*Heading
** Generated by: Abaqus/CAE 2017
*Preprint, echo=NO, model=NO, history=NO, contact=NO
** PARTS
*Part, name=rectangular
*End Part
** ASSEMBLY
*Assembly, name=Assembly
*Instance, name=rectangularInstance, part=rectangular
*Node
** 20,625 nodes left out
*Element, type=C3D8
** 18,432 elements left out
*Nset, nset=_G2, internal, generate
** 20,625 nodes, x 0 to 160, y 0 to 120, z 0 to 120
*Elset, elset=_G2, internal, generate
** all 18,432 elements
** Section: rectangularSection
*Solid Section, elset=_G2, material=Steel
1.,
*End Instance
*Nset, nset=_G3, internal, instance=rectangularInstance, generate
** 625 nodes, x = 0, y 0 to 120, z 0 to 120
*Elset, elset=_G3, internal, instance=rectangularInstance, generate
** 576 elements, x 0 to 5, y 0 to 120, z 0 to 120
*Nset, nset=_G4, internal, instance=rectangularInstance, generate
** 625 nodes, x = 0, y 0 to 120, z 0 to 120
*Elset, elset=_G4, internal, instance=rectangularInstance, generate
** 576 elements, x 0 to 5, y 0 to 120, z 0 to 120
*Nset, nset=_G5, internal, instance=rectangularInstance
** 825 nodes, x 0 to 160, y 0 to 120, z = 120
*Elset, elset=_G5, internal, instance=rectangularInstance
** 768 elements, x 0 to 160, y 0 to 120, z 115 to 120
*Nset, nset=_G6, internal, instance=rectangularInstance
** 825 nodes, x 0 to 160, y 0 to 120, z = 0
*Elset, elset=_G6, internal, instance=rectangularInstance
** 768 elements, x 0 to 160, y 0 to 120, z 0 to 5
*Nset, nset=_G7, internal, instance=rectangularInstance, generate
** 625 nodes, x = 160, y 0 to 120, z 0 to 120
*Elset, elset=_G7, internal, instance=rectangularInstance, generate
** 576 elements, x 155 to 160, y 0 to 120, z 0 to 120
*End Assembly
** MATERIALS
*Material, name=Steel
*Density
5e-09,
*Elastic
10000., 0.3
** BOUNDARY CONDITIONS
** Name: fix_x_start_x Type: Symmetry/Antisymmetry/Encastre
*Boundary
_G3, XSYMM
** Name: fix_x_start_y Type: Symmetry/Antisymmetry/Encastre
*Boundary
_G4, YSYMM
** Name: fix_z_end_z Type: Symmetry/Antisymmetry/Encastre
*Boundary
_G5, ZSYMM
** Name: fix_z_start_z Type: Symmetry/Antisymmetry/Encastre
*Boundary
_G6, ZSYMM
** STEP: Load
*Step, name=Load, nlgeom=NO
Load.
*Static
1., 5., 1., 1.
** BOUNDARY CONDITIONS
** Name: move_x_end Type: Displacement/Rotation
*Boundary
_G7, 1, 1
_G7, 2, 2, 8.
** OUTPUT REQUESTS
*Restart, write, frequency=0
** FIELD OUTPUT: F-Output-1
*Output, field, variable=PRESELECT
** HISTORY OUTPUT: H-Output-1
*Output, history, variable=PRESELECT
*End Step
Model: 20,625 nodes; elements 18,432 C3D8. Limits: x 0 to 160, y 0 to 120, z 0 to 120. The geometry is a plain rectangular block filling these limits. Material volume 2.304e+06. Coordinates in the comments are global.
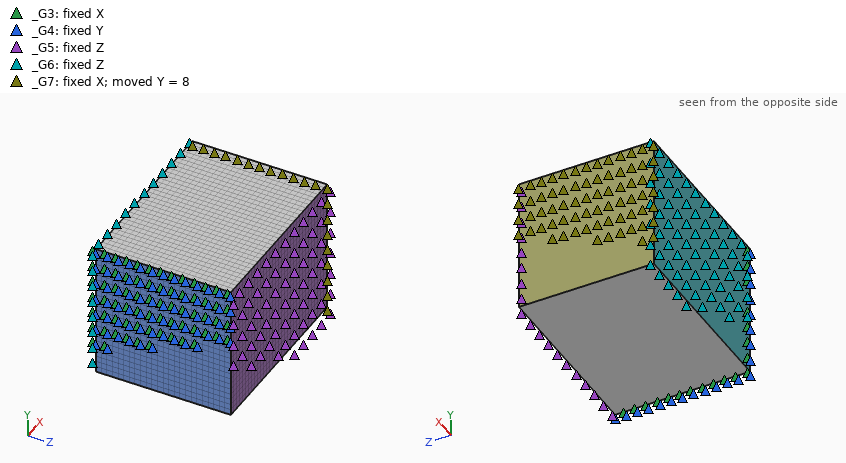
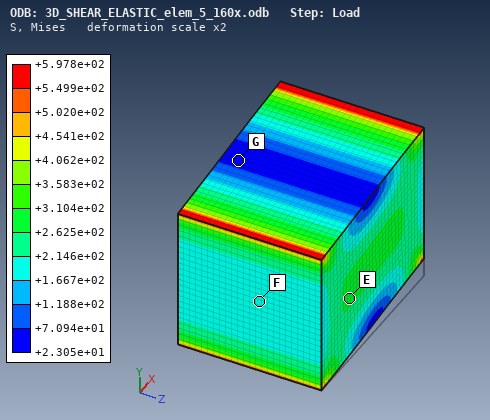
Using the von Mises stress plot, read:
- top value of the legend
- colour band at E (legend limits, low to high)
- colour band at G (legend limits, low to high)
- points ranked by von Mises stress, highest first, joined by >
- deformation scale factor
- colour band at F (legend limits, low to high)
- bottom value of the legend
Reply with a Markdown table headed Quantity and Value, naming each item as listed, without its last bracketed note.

| Quantity | Value |
|---|---|
| top value of the legend | +5.978e+02 |
| colour band at E | +2.625e+02 to +3.104e+02 |
| colour band at G | +2.305e+01 to +7.094e+01 |
| points ranked by von Mises stress, highest first, joined by > | E > F > G |
| deformation scale factor | 2 |
| colour band at F | +1.667e+02 to +2.146e+02 |
| bottom value of the legend | +2.305e+01 |
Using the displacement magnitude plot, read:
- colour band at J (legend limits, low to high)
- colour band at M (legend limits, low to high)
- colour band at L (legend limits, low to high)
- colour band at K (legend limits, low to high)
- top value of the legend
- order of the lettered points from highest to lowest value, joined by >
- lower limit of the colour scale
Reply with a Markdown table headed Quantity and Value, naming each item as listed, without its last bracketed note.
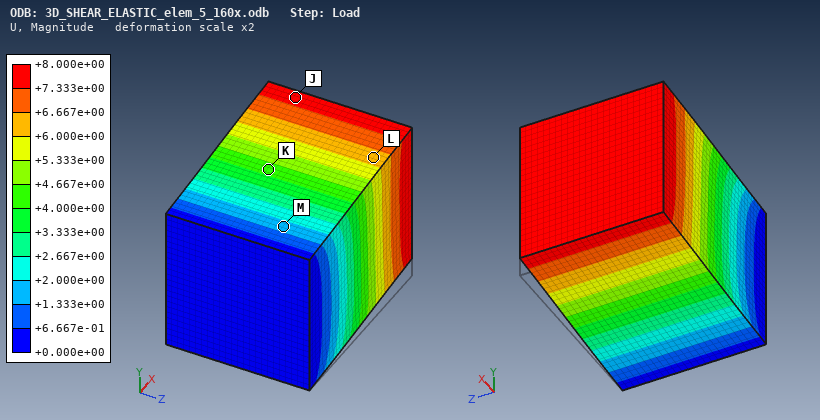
| Quantity | Value |
|---|---|
| colour band at J | +7.333e+00 to +8.000e+00 |
| colour band at M | +1.333e+00 to +2.000e+00 |
| colour band at L | +6.000e+00 to +6.667e+00 |
| colour band at K | +4.000e+00 to +4.667e+00 |
| top value of the legend | +8.000e+00 |
| order of the lettered points from highest to lowest value, joined by > | J > L > K > M |
| lower limit of the colour scale | +0.000e+00 |
